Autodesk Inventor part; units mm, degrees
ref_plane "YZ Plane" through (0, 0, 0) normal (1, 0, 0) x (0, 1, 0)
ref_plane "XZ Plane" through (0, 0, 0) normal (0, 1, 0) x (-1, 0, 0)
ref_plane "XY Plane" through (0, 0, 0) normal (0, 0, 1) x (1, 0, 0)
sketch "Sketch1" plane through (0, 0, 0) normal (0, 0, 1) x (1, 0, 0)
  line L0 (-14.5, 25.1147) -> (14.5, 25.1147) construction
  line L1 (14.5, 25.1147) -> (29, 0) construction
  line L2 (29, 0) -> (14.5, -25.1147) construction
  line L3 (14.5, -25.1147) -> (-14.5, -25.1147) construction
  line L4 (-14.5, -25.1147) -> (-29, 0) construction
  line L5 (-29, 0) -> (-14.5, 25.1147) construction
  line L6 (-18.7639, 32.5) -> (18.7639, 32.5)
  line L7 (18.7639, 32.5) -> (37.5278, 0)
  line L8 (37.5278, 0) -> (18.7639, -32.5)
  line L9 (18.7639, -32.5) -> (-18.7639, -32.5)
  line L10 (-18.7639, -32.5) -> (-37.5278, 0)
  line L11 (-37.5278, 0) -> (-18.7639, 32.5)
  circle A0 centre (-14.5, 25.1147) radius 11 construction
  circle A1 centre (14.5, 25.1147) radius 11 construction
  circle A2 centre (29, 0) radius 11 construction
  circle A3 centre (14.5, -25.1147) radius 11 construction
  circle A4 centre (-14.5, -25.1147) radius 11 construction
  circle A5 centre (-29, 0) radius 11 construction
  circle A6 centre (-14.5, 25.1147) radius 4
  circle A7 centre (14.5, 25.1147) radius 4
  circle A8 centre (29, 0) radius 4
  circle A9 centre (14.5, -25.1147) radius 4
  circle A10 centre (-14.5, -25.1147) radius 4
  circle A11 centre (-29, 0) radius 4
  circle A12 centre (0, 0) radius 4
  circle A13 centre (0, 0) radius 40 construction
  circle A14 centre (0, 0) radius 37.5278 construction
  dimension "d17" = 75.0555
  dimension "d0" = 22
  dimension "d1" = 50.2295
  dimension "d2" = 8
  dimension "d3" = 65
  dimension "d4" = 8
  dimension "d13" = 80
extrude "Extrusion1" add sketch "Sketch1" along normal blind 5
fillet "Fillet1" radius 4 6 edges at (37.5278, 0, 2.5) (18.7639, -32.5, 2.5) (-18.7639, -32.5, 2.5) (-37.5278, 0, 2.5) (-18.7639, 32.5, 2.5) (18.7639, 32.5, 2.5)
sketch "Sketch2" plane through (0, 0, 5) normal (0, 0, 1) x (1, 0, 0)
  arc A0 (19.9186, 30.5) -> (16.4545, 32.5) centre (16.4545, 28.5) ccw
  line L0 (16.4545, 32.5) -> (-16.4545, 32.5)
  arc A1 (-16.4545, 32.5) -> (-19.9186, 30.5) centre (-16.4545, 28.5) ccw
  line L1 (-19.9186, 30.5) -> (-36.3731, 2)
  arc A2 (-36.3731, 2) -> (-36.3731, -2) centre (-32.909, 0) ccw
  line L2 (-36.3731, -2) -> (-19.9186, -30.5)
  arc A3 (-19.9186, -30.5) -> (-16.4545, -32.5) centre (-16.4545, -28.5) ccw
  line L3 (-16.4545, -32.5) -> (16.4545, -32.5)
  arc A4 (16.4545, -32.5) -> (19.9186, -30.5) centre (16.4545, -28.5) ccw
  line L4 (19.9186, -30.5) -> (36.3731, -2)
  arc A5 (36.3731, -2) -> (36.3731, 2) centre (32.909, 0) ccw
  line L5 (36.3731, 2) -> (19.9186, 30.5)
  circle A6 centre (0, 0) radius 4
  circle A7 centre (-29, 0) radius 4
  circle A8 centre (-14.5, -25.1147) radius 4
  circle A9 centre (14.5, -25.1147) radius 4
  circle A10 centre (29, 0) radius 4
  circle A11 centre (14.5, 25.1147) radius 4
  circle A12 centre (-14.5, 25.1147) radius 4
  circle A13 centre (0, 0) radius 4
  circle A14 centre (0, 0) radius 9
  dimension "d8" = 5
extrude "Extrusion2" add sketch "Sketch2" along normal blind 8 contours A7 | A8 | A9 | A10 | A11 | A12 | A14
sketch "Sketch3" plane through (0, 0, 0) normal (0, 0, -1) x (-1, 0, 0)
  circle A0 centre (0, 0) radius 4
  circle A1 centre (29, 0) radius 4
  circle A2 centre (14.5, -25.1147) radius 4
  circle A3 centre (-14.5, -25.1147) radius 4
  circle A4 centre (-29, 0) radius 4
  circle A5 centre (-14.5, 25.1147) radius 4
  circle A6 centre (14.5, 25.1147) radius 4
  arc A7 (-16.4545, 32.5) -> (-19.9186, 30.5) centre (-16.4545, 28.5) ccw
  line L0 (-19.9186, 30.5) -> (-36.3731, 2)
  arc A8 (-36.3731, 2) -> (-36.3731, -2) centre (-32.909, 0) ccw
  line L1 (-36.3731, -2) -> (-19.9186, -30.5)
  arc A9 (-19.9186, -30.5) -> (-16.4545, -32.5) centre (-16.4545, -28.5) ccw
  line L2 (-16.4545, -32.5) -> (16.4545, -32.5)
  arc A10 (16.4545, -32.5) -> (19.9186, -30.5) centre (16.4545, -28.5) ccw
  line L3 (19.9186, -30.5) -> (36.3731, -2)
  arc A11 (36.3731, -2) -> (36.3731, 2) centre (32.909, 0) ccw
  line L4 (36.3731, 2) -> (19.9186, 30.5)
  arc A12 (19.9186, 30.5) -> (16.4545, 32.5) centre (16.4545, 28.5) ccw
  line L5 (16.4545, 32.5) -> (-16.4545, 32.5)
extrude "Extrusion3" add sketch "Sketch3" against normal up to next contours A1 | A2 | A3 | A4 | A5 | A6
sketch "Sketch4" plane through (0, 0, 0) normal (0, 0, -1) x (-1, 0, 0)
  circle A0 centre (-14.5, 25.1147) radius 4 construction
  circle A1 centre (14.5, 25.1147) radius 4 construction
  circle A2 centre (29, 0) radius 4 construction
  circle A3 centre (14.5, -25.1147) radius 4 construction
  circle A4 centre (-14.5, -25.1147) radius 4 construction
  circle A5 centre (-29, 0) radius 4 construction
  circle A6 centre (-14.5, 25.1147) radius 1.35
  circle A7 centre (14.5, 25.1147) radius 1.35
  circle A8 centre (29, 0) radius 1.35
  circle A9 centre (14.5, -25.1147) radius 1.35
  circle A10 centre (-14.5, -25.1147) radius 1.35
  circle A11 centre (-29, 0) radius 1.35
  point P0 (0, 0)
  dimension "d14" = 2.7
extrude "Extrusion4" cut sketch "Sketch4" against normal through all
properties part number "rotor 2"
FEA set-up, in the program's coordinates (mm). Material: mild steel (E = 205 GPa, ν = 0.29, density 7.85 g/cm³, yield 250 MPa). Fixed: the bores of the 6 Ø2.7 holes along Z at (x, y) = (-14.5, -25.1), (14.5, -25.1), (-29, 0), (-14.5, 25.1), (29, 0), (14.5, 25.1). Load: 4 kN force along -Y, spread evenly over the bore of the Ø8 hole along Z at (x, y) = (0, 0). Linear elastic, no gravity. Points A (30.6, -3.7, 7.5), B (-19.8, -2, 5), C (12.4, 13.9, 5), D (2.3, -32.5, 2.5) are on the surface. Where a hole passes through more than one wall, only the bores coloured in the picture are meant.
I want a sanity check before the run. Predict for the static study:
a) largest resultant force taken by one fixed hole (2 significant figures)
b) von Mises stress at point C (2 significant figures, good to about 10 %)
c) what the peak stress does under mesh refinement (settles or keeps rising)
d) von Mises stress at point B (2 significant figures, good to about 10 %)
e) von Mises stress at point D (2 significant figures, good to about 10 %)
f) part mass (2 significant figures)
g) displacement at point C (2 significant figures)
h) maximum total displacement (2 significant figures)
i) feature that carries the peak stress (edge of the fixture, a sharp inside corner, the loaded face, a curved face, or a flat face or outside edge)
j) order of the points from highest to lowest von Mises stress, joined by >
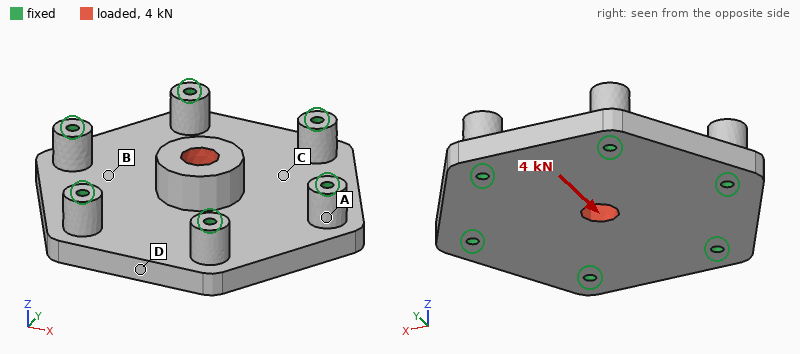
910 N
19 MPa
keeps rising
12 MPa
8.6 MPa
170 g
1.5 µm
7.4 µm
edge of the fixture
C > B > D > A
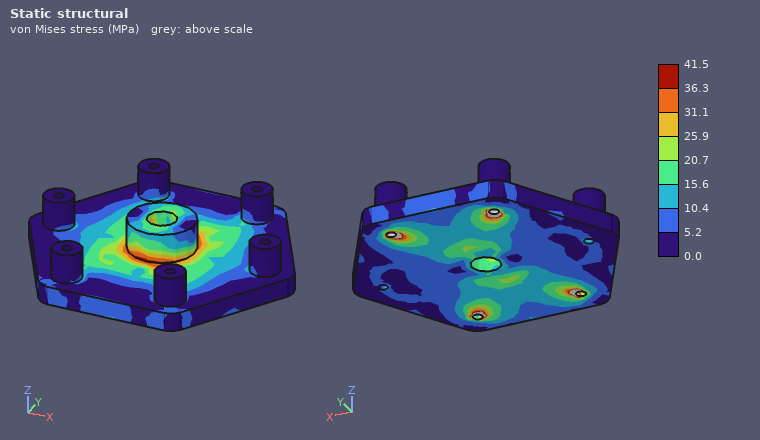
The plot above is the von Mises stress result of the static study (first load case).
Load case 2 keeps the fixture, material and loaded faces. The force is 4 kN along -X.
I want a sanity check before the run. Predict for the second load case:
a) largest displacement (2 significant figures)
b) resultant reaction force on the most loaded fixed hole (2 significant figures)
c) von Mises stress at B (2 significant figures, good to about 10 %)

7.4 µm
1.0 kN
17 MPa
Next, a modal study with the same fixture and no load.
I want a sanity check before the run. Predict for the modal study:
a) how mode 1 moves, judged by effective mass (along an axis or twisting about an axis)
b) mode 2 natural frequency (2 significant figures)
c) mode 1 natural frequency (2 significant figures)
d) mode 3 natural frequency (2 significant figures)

along Z
20 kHz
11 kHz
20 kHz
